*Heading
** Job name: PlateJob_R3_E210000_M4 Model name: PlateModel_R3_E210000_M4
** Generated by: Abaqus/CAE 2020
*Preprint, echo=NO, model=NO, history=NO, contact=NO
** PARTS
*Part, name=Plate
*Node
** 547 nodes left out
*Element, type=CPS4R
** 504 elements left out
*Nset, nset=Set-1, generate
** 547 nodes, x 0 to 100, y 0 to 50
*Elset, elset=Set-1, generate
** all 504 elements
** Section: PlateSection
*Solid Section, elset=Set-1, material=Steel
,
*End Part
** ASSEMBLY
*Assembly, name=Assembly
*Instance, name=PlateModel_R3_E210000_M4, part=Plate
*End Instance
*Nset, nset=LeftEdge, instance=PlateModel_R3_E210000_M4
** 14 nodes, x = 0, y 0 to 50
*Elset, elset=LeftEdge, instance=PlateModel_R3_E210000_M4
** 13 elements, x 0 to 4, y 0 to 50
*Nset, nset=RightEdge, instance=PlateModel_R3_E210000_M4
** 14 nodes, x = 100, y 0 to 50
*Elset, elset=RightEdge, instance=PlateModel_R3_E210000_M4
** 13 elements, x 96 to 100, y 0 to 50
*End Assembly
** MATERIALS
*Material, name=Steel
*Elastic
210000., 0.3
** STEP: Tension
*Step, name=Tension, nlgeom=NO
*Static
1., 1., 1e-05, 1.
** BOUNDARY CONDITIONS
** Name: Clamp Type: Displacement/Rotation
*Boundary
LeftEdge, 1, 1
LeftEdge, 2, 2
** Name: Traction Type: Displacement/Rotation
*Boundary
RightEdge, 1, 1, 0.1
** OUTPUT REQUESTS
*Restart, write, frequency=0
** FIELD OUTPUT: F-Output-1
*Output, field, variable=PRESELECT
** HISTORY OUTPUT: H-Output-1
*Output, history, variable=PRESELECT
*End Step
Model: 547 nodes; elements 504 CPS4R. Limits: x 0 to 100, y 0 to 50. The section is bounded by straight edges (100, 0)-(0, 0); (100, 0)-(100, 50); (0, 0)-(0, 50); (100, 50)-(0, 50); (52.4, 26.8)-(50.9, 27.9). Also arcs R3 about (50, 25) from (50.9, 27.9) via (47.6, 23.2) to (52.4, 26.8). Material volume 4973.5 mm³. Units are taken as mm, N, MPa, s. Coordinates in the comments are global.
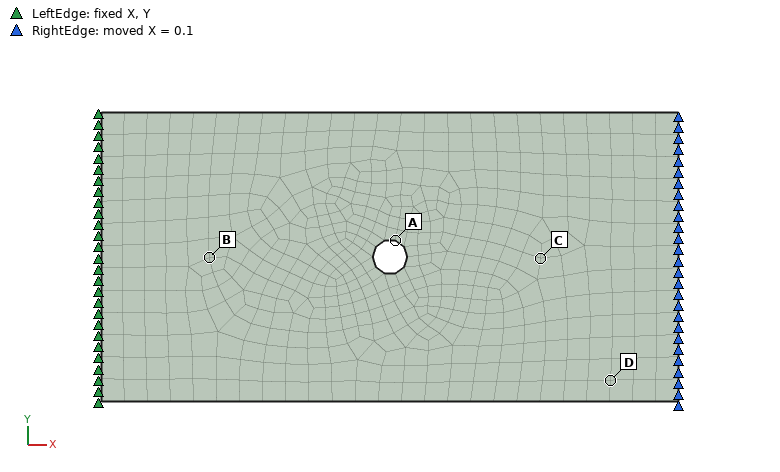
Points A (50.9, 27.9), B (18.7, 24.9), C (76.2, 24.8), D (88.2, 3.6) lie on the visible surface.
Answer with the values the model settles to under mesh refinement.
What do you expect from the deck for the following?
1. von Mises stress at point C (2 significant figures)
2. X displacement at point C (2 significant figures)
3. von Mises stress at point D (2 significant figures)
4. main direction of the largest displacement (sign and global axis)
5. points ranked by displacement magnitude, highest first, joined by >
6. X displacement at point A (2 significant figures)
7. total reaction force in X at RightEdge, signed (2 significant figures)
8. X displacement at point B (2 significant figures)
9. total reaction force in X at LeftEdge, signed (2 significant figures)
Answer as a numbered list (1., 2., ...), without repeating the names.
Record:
1. 200 MPa
2. 0.077 mm
3. 210 MPa
4. +X
5. D > C > A > B
6. 0.052 mm
7. 10000 N
8. 0.017 mm
9. -10000 N
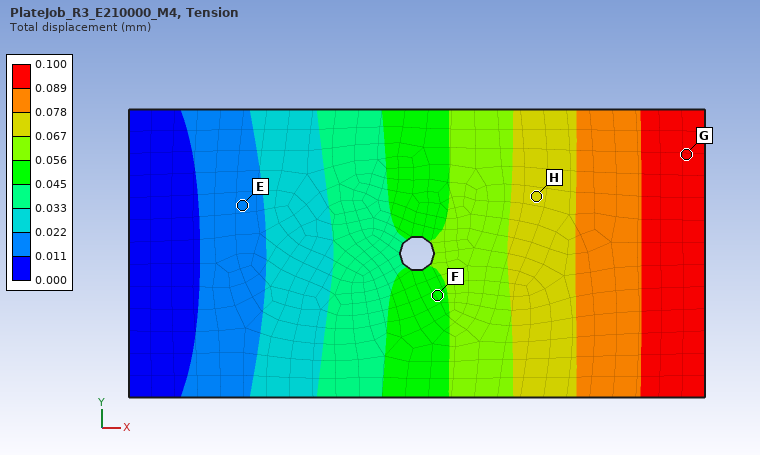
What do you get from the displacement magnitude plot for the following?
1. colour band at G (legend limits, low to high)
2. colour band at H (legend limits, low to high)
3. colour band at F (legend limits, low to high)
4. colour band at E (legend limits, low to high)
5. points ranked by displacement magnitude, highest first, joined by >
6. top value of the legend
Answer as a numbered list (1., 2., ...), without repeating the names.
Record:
1. 0.089 to 0.100 mm
2. 0.067 to 0.078 mm
3. 0.045 to 0.056 mm
4. 0.011 to 0.022 mm
5. G > H > F > E
6. 0.100 mm
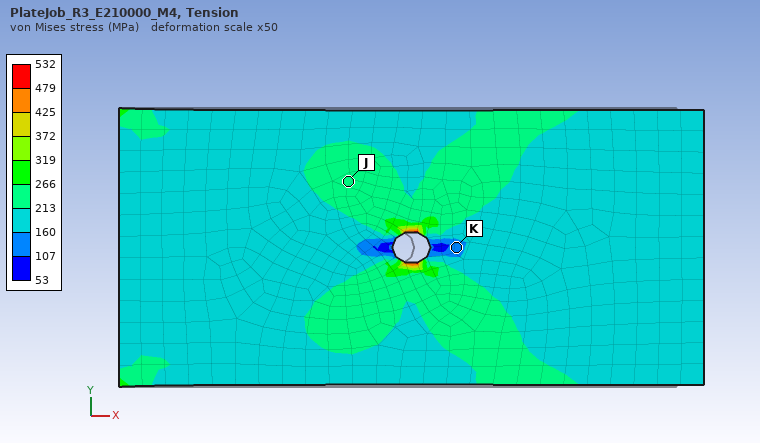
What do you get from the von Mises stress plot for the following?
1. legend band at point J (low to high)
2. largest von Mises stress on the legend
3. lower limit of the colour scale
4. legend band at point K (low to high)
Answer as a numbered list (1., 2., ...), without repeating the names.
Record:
1. 213 to 266 MPa
2. 532 MPa
3. 53 MPa
4. 107 to 160 MPa
